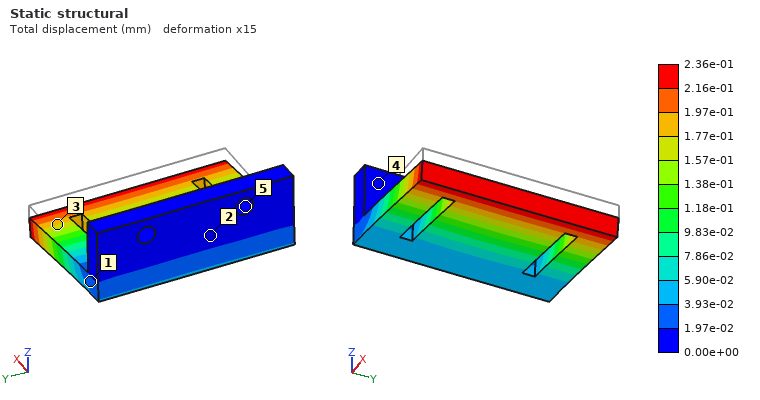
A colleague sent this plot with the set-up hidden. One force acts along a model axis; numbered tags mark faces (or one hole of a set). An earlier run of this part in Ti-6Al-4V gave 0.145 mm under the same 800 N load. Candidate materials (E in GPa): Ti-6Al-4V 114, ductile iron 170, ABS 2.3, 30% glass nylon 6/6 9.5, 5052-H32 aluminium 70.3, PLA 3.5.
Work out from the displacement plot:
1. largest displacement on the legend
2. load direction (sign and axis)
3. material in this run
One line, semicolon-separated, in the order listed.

2.36e-01 mm; -Z; 5052-H32 aluminium
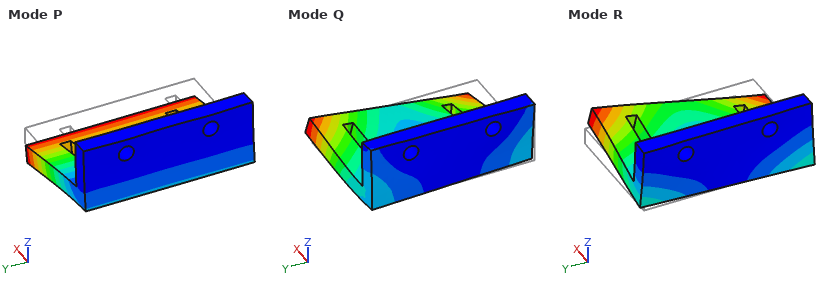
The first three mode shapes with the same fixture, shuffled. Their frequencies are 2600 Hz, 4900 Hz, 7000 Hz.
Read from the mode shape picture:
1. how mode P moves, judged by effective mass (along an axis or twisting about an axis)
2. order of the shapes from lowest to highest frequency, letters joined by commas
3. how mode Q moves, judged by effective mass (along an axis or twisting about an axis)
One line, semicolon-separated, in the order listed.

along Z; P, R, Q; along Y
